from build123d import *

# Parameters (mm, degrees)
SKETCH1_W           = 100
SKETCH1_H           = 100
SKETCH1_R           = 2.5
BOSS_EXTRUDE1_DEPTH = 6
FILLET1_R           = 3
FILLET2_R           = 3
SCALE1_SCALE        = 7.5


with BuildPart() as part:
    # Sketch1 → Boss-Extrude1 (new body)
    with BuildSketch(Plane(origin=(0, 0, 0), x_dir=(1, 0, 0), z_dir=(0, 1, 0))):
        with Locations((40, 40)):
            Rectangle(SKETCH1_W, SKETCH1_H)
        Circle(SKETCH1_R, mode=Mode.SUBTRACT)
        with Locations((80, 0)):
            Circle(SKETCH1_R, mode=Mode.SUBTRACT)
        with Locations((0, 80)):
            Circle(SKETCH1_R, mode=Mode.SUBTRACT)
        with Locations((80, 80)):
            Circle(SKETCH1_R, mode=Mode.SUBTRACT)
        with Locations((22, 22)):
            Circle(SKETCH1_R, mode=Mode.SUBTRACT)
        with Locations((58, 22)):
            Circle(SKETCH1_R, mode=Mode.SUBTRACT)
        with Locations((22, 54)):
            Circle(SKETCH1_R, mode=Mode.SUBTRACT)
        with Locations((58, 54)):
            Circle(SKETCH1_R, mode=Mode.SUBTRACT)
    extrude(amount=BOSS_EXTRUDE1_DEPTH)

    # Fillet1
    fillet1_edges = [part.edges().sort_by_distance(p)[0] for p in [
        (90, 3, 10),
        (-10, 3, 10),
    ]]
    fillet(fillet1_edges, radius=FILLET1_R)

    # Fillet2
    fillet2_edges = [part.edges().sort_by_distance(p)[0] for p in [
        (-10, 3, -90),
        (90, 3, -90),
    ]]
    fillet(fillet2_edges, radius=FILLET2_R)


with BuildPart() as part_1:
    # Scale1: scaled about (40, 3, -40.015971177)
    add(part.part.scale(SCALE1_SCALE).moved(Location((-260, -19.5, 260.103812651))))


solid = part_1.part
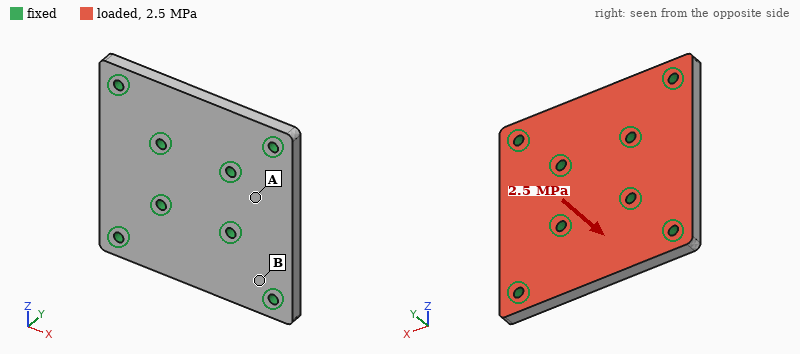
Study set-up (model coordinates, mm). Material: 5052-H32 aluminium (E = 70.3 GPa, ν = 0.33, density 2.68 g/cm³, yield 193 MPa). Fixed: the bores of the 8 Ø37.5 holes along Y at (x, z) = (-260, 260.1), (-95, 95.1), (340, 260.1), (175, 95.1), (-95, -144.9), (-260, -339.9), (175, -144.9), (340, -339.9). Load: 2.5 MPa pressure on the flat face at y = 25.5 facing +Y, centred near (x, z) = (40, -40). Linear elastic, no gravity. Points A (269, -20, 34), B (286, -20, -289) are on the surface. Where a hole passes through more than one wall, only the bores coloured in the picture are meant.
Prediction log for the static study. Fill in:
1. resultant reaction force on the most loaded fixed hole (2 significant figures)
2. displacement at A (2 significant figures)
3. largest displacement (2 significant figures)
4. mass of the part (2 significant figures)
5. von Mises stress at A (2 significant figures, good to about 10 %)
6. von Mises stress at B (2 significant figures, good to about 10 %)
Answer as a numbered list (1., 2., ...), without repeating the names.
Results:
1. 210 kN
2. 0.24 mm
3. 1.0 mm
4. 67 kg
5. 22 MPa
6. 70 MPa
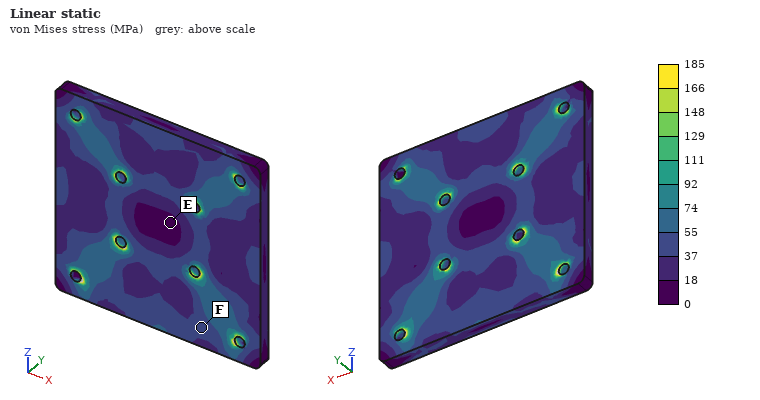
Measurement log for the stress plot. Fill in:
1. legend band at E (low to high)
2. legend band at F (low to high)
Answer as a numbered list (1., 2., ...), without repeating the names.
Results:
1. 0 to 18 MPa
2. 37 to 55 MPa
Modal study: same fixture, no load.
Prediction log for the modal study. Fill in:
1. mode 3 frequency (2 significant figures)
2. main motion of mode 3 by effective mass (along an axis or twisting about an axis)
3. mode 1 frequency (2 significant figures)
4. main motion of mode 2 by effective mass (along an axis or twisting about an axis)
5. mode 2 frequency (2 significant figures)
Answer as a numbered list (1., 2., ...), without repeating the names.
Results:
1. 1000 Hz
2. twisting about Z
3. 880 Hz
4. twisting about X
5. 970 Hz
